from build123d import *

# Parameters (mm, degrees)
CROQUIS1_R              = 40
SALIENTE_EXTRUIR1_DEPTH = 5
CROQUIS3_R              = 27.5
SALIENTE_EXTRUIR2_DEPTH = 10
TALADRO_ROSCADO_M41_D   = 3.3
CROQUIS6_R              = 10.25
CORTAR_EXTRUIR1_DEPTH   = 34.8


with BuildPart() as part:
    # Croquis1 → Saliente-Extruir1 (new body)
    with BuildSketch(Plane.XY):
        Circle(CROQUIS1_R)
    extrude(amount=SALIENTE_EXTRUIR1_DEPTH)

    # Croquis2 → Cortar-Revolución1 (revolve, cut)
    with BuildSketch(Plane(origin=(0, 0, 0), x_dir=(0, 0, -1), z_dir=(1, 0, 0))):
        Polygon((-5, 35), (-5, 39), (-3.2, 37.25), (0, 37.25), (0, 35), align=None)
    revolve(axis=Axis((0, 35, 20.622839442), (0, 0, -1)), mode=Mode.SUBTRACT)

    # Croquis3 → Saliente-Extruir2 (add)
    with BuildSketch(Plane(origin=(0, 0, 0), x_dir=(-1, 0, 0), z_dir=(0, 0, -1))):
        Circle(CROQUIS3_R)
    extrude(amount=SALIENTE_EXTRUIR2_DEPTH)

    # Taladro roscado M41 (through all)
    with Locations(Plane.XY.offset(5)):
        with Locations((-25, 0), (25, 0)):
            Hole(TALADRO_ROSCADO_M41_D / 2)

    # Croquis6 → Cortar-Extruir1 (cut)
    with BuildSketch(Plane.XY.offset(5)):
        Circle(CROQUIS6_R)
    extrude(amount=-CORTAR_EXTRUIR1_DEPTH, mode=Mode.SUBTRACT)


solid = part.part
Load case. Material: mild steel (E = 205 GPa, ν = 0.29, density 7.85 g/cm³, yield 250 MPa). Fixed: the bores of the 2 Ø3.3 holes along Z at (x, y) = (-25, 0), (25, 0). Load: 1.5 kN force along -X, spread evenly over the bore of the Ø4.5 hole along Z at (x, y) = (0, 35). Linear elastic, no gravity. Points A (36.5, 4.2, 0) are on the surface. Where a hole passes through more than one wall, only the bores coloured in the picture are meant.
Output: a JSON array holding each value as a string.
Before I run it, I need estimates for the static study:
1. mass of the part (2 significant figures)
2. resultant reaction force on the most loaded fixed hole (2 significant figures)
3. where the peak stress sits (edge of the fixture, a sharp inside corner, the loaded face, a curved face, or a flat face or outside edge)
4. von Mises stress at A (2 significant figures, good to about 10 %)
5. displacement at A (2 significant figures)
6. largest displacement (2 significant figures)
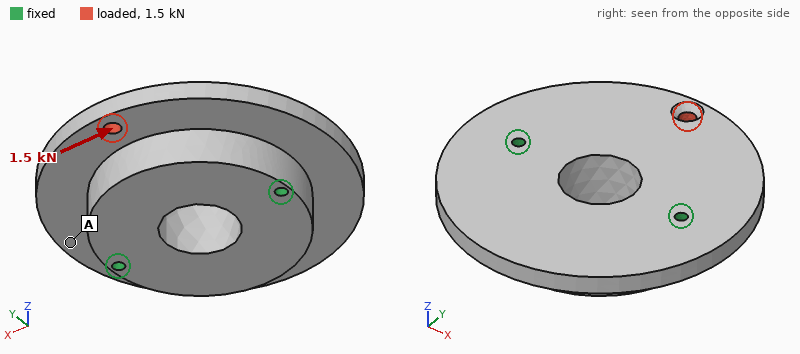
["340 g", "1.3 kN", "the loaded face", "3.7 MPa", "0.66 µm", "3.6 µm"]
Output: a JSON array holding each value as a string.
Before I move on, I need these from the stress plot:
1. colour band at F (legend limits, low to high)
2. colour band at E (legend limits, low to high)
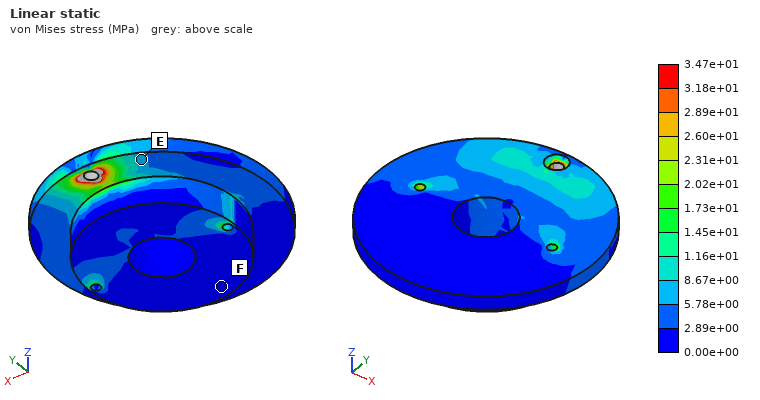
["0.00e+00 to 2.89e+00 MPa", "5.78e+00 to 8.67e+00 MPa"]
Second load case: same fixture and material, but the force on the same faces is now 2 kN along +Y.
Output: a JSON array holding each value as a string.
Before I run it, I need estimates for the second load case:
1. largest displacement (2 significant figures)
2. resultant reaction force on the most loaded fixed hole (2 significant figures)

["5.2 µm", "1.1 kN"]
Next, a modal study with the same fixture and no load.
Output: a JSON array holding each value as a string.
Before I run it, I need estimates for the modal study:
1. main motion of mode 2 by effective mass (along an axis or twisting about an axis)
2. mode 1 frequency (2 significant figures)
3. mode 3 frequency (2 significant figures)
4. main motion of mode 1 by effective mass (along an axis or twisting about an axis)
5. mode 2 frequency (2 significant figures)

["along Z", "6300 Hz", "12 kHz", "twisting about X", "8300 Hz"]
